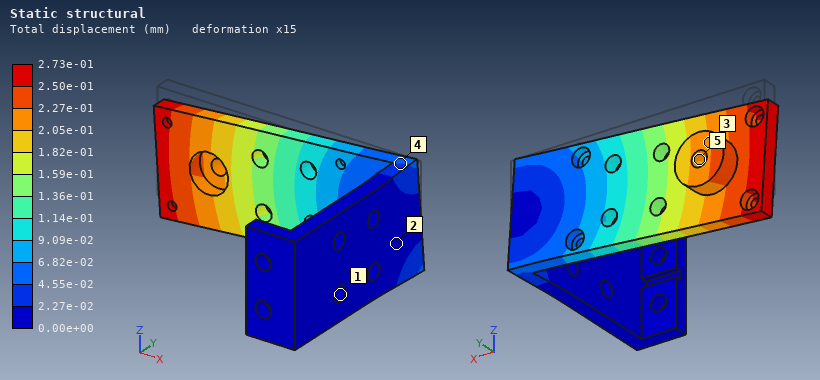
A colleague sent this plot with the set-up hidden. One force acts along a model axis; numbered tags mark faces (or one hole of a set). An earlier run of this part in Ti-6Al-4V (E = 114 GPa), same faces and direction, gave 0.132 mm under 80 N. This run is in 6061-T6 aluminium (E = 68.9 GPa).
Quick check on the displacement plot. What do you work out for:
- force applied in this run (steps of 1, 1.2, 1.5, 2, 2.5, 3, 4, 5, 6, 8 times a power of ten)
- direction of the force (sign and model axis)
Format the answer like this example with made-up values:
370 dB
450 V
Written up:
100 N
-Z
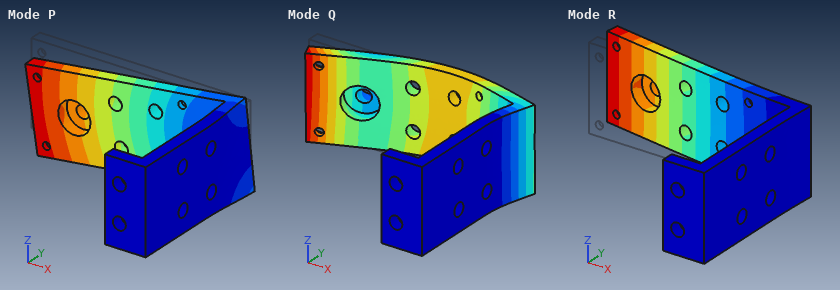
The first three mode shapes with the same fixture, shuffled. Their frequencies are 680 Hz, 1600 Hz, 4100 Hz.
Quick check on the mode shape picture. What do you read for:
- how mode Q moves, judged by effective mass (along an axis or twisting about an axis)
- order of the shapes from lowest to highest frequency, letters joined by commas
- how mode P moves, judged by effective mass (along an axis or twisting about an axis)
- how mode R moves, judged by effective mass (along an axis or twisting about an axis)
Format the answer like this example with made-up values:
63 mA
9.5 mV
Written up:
along X
R, P, Q
along Z
along Y
